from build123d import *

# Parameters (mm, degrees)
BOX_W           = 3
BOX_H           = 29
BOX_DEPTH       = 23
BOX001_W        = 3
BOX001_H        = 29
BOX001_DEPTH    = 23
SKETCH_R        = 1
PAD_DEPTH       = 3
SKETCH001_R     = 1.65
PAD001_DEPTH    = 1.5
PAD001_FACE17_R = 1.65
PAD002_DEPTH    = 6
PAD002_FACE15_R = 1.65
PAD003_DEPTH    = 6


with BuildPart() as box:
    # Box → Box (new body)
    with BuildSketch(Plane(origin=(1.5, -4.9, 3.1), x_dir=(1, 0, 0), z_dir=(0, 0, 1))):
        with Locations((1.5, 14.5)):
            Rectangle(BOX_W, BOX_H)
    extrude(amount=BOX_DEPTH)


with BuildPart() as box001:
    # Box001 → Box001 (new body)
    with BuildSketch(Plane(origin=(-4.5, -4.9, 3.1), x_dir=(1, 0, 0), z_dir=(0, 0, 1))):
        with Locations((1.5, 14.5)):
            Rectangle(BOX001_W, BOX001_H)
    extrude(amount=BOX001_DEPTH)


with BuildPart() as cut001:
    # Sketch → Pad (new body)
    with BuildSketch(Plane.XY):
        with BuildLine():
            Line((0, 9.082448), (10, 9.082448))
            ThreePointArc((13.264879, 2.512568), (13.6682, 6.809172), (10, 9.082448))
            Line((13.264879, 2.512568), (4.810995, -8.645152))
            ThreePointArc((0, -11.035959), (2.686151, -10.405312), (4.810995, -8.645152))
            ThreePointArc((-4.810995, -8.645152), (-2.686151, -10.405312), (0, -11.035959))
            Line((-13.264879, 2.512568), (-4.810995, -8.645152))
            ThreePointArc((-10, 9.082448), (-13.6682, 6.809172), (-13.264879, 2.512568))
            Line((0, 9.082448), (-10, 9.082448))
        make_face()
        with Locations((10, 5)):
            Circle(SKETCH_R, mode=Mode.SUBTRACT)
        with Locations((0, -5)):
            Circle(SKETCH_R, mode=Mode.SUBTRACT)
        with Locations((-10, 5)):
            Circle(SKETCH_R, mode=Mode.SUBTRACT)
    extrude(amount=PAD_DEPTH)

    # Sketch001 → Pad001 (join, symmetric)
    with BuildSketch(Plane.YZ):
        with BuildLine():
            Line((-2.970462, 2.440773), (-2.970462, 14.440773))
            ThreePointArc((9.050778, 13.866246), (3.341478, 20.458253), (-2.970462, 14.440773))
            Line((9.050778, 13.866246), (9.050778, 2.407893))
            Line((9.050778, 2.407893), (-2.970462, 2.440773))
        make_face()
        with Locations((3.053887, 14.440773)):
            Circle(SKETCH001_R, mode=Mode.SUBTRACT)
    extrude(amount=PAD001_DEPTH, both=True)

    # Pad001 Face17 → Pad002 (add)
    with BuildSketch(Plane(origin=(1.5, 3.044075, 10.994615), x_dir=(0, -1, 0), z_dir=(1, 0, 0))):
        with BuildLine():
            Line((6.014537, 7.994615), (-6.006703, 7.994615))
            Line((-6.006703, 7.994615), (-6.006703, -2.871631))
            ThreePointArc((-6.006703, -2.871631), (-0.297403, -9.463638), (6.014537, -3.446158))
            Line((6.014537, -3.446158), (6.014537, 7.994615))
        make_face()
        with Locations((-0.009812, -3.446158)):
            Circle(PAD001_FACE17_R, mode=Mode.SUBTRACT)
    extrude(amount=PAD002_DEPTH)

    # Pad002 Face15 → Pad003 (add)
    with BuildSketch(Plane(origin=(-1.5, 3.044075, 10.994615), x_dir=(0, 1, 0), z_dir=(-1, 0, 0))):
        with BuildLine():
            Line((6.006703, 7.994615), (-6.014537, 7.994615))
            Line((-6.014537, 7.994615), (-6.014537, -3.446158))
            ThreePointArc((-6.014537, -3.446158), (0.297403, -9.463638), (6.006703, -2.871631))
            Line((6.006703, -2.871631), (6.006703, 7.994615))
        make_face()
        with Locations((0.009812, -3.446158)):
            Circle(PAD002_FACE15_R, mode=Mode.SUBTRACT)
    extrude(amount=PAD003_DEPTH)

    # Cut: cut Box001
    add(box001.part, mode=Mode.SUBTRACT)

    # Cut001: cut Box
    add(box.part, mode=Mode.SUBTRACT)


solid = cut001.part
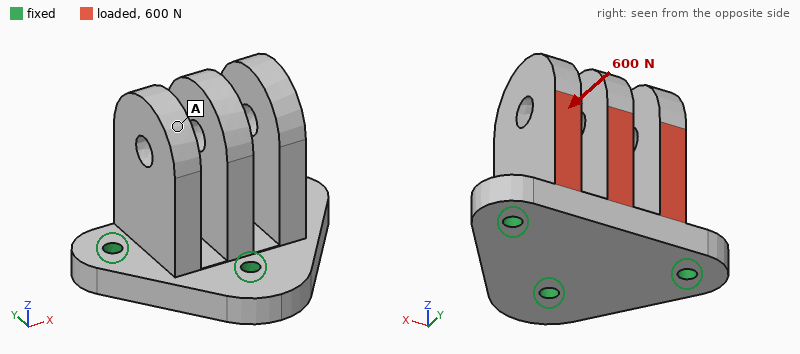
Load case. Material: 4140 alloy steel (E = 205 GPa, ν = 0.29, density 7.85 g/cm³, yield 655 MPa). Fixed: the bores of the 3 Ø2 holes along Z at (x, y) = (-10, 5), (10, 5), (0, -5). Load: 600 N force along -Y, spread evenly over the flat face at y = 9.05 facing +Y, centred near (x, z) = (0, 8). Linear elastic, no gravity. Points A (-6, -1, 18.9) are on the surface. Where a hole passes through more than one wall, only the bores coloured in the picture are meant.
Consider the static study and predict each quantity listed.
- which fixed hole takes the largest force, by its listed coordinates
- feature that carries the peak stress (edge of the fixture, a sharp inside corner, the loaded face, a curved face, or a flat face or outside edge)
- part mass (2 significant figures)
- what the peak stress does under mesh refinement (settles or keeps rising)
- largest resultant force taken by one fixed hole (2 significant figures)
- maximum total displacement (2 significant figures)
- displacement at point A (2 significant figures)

(0, -5)
edge of the fixture
22 g
keeps rising
430 N
9.1 µm
8.3 µm
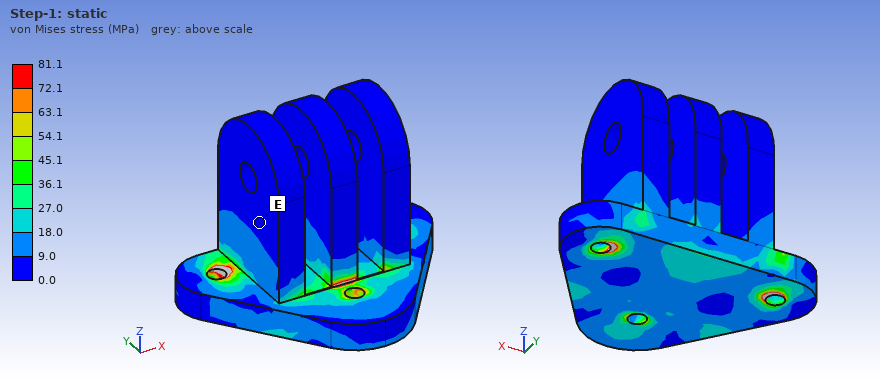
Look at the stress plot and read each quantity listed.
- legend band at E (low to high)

0.0 to 9.0 MPa
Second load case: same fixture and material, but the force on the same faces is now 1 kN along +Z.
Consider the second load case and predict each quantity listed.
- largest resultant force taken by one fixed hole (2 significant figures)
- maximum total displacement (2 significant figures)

570 N
20 µm
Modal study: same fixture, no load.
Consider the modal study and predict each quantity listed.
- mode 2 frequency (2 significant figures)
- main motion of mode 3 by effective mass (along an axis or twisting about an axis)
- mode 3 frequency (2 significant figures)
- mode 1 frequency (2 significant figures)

7800 Hz
along X
8400 Hz
7200 Hz
